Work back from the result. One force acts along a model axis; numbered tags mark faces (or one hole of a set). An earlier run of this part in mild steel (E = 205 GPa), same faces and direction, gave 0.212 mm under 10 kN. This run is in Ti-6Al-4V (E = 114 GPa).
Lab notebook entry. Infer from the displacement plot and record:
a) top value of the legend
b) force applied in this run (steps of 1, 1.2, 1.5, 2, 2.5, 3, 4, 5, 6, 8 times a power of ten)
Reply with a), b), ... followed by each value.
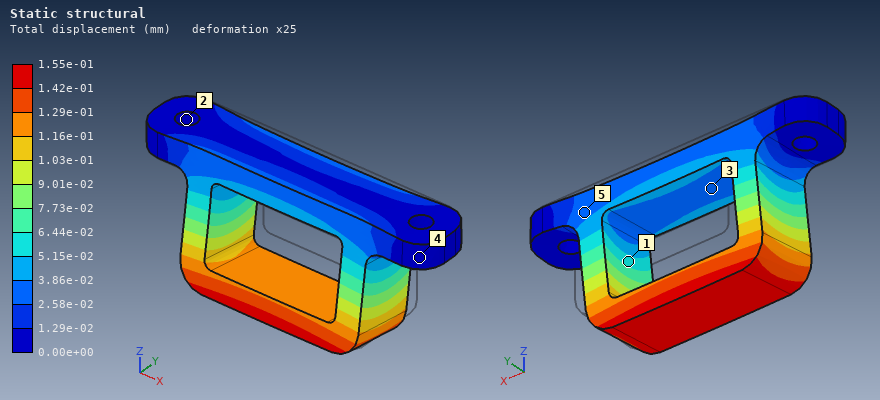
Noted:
a) 1.55e-01 mm
b) 4 kN
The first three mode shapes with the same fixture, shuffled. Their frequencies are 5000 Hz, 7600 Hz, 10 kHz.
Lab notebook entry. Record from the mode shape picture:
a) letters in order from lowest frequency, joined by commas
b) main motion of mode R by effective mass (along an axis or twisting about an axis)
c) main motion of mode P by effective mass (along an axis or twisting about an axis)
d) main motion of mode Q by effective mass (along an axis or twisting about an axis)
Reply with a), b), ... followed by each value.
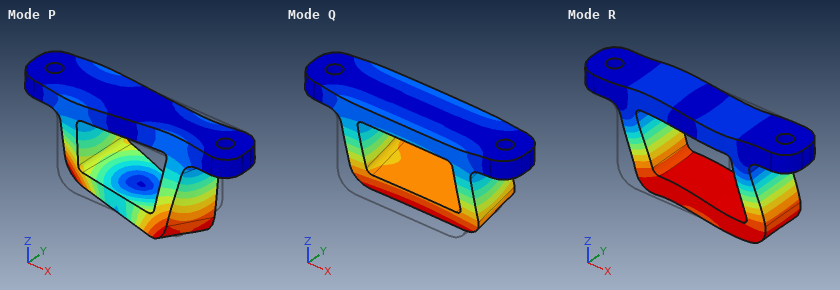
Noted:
a) Q, R, P
b) along X
c) twisting about Z
d) along Y
